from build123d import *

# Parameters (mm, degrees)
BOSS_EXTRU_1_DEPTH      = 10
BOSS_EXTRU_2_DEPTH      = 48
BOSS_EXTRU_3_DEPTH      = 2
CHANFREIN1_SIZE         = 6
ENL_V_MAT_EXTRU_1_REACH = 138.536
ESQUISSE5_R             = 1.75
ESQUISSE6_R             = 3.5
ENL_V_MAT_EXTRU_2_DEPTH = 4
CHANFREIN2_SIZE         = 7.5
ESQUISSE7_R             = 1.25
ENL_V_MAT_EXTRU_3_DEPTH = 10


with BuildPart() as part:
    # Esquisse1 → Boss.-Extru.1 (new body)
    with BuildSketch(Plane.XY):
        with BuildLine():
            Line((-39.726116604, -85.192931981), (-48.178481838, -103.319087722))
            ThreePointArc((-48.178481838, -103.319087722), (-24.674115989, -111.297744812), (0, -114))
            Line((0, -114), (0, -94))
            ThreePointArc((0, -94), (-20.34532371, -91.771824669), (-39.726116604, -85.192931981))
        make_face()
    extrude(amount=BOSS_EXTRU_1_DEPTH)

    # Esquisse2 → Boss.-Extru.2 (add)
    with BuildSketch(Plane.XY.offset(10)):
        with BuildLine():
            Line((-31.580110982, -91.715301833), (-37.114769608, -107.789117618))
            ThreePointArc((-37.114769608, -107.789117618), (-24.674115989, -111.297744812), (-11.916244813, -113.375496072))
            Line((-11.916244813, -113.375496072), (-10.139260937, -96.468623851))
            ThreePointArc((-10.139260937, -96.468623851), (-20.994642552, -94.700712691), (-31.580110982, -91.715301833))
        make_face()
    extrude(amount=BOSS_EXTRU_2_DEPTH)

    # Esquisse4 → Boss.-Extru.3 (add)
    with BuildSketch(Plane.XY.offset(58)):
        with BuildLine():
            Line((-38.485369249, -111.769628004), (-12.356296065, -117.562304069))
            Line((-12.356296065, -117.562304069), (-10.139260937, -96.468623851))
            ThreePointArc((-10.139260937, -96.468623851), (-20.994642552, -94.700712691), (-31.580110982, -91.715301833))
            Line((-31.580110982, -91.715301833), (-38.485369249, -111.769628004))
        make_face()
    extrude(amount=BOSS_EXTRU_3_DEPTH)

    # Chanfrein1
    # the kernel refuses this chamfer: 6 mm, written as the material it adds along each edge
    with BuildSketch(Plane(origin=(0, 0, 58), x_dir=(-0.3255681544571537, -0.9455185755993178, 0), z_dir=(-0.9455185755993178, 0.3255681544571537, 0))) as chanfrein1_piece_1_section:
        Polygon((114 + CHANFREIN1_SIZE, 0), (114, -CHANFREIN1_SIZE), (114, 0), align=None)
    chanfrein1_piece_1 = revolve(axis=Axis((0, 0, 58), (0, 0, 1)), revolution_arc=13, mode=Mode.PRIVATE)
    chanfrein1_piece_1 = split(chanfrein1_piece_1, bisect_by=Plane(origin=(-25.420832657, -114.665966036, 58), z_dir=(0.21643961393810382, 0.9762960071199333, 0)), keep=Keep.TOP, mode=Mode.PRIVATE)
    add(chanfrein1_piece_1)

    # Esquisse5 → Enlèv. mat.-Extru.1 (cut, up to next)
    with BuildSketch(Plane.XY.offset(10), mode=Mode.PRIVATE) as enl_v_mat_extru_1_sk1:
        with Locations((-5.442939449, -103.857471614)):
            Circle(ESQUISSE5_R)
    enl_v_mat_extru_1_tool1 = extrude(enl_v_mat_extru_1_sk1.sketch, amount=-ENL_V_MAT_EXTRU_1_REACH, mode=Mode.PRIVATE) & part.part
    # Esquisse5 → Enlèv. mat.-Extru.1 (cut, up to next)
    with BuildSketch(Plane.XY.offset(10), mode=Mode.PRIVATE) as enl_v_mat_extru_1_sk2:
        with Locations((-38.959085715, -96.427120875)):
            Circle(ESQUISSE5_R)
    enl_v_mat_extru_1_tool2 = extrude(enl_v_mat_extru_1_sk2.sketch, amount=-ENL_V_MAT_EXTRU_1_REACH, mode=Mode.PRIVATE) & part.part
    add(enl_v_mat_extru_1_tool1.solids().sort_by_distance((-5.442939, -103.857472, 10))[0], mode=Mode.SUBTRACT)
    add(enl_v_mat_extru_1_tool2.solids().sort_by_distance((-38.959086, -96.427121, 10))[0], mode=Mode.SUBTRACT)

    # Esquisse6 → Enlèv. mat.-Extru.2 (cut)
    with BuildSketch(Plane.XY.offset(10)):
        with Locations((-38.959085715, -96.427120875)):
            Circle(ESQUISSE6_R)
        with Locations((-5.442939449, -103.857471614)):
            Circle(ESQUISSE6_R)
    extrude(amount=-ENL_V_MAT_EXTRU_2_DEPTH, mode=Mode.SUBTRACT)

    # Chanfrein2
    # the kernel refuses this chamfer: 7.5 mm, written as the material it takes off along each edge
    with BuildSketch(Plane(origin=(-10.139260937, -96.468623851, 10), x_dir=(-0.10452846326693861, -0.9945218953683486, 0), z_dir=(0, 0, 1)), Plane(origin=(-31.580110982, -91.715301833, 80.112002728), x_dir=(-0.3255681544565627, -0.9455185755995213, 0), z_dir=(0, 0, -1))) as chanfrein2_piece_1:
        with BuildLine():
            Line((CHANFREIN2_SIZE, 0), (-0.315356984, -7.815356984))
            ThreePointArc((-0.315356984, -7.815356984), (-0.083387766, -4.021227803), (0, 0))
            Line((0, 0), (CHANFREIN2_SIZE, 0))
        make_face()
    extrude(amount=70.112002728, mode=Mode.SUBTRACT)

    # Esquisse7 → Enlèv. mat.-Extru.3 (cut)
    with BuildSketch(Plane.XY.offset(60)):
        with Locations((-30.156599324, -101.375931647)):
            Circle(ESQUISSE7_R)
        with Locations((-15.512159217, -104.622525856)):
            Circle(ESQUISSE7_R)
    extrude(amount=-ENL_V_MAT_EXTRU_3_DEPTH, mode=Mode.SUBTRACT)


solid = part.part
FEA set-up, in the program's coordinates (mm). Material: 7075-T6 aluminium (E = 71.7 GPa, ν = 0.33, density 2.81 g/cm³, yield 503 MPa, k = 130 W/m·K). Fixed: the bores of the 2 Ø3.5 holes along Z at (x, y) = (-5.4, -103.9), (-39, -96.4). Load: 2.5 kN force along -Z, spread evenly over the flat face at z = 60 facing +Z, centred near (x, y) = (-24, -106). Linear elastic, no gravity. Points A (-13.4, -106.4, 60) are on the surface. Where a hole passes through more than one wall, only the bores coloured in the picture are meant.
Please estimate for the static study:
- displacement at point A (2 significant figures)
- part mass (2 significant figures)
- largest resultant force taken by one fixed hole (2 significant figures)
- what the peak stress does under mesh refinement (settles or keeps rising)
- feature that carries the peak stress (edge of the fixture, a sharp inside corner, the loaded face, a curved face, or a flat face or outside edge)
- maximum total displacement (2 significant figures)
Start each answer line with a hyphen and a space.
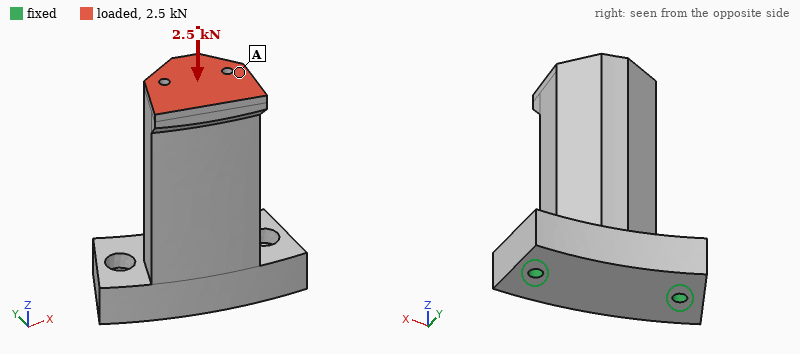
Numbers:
- 85 µm
- 75 g
- 1.4 kN
- keeps rising
- edge of the fixture
- 91 µm
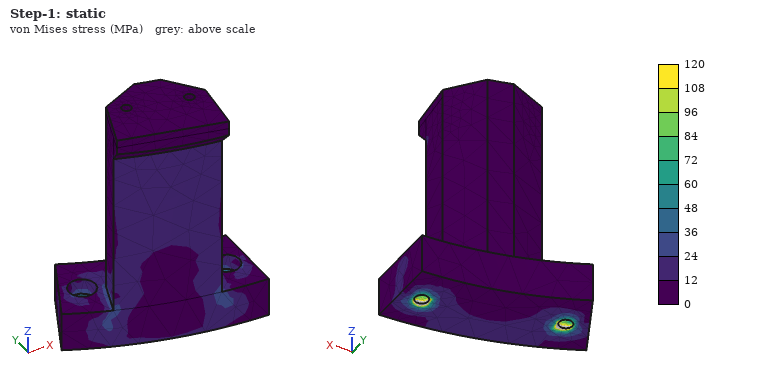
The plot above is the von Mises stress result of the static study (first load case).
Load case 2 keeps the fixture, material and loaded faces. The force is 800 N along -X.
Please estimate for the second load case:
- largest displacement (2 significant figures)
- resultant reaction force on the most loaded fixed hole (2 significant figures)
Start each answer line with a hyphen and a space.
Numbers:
- 0.10 mm
- 1.5 kN
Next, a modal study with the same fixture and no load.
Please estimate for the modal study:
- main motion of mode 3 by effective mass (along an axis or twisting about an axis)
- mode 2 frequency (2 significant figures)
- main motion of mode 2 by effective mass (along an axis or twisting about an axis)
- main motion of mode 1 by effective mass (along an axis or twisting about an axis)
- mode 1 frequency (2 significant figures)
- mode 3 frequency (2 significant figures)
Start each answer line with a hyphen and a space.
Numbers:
- along Z
- 4300 Hz
- along X
- along Y
- 1800 Hz
- 11 kHz
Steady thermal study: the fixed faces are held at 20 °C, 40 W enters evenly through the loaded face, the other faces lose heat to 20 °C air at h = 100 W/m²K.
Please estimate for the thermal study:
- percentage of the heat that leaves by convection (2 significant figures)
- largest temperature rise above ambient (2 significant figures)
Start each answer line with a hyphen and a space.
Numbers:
- 31 %
- 46 K
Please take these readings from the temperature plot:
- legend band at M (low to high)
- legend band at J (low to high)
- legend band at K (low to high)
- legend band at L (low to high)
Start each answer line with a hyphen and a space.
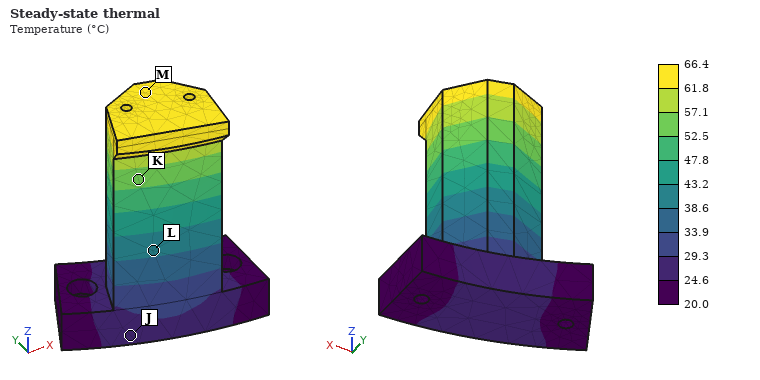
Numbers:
- 61.8 to 66.4 °C
- 24.6 to 29.3 °C
- 52.5 to 57.1 °C
- 38.6 to 43.2 °C
